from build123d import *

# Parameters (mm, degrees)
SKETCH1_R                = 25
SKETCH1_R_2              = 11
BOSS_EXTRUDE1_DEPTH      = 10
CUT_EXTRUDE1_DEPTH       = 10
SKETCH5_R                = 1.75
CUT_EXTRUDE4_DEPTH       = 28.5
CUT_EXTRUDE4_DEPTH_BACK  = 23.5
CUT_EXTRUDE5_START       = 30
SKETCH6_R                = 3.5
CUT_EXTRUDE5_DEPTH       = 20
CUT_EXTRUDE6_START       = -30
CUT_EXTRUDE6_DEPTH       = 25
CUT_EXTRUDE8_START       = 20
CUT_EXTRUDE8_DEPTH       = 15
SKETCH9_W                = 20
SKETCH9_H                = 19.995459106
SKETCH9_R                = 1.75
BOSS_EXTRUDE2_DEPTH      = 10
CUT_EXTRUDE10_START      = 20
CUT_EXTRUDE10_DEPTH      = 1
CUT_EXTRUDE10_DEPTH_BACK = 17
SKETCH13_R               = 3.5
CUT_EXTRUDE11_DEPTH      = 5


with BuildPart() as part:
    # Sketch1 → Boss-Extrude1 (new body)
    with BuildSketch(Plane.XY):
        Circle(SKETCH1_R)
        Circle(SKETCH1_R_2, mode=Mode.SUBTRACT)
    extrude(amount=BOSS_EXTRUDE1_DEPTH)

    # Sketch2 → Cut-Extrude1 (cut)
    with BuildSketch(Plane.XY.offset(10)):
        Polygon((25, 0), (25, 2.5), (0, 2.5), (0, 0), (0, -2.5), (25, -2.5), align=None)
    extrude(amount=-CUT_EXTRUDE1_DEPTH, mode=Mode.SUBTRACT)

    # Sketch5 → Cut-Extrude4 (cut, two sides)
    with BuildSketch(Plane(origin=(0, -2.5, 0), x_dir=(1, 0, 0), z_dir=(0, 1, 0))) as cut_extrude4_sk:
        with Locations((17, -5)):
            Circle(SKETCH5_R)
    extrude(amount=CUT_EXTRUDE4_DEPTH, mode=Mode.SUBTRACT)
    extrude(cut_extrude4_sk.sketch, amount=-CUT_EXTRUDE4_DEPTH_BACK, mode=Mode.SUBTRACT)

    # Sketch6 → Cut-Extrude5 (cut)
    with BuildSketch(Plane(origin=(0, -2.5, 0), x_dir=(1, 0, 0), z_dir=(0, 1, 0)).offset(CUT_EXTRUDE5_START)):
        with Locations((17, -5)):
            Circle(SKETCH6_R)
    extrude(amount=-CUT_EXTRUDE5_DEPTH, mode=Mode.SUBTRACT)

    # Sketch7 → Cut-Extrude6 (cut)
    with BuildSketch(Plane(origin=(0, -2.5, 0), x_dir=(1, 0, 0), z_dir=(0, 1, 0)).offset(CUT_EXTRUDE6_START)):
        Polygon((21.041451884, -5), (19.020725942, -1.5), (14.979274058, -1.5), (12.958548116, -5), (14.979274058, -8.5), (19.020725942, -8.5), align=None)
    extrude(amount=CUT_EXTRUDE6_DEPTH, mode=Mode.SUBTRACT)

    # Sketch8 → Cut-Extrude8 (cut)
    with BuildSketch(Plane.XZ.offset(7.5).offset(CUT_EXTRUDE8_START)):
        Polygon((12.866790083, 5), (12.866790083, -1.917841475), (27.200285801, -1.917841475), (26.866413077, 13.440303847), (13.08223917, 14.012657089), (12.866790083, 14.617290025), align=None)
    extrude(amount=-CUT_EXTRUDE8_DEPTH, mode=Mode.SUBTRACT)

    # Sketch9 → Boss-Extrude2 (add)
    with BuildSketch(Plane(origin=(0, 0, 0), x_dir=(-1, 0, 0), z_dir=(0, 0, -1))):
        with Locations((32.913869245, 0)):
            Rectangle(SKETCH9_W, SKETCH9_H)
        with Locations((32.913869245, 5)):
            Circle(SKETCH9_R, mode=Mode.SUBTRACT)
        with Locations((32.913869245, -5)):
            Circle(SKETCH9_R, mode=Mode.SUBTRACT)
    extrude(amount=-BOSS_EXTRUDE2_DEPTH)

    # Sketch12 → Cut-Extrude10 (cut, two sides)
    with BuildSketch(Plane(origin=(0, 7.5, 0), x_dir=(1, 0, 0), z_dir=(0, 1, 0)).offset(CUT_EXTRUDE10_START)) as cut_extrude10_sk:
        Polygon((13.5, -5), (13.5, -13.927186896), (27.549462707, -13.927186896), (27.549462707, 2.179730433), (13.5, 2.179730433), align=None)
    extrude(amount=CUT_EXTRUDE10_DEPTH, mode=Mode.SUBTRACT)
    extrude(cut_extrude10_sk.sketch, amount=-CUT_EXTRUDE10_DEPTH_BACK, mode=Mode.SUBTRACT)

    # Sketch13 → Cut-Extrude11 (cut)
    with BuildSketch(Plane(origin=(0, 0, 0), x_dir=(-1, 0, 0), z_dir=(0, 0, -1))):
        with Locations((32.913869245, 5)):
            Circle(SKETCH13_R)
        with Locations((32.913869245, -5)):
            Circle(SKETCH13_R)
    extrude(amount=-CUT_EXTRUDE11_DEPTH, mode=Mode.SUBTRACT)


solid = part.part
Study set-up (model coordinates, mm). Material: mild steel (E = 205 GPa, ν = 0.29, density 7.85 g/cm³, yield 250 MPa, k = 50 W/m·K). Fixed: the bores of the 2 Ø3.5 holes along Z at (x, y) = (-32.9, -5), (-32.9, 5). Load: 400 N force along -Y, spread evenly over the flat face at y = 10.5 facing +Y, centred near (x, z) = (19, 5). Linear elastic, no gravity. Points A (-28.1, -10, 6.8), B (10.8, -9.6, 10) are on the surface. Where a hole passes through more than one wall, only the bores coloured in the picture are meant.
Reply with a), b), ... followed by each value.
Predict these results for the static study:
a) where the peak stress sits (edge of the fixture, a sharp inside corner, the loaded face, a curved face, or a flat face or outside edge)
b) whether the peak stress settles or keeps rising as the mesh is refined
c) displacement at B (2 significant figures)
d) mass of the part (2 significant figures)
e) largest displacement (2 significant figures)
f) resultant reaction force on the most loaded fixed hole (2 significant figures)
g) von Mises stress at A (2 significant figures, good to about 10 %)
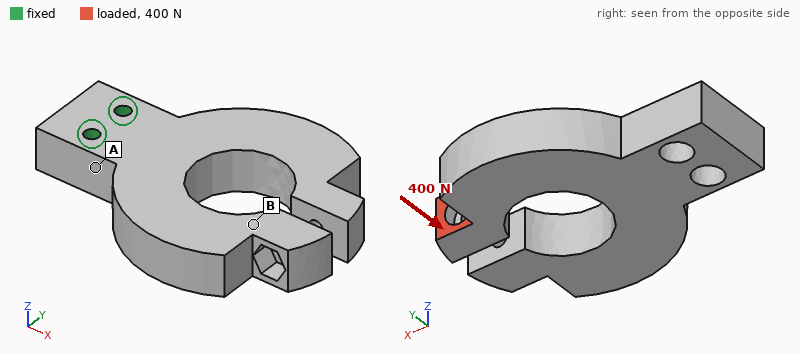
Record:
a) edge of the fixture
b) keeps rising
c) 12 µm
d) 130 g
e) 54 µm
f) 1.7 kN
g) 30 MPa
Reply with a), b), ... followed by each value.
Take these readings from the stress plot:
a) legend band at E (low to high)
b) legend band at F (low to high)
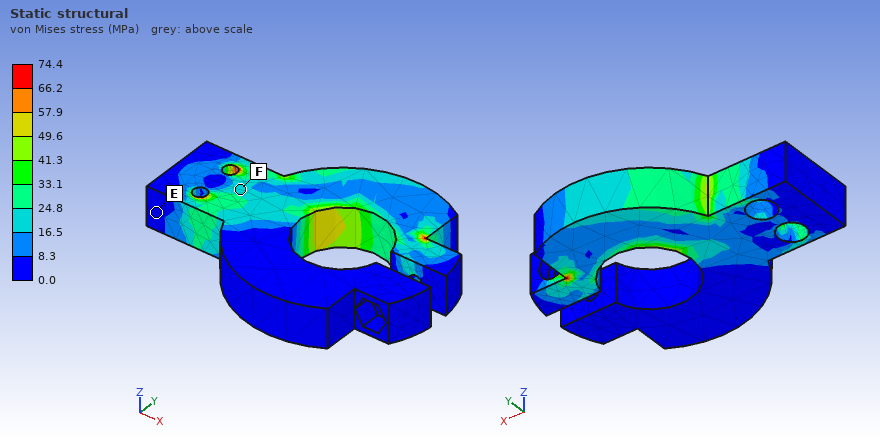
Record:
a) 0.0 to 8.3 MPa
b) 16.5 to 24.8 MPa
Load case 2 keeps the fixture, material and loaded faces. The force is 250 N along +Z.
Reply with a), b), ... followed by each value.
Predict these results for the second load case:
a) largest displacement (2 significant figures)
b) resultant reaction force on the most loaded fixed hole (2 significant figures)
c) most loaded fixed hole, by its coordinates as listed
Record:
a) 90 µm
b) 320 N
c) (-32.9, 5)
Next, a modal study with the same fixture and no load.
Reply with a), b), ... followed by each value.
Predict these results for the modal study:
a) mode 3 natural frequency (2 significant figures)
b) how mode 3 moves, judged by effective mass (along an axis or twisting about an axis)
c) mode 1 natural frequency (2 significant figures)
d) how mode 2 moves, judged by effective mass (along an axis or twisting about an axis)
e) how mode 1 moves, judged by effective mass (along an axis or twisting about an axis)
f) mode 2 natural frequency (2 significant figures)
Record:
a) 3300 Hz
b) along Y
c) 1700 Hz
d) along Y
e) along Z
f) 3100 Hz
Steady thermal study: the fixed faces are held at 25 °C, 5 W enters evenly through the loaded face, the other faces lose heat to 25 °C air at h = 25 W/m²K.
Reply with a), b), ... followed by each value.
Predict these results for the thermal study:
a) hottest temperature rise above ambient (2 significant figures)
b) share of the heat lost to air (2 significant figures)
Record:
a) 48 K
b) 34 %
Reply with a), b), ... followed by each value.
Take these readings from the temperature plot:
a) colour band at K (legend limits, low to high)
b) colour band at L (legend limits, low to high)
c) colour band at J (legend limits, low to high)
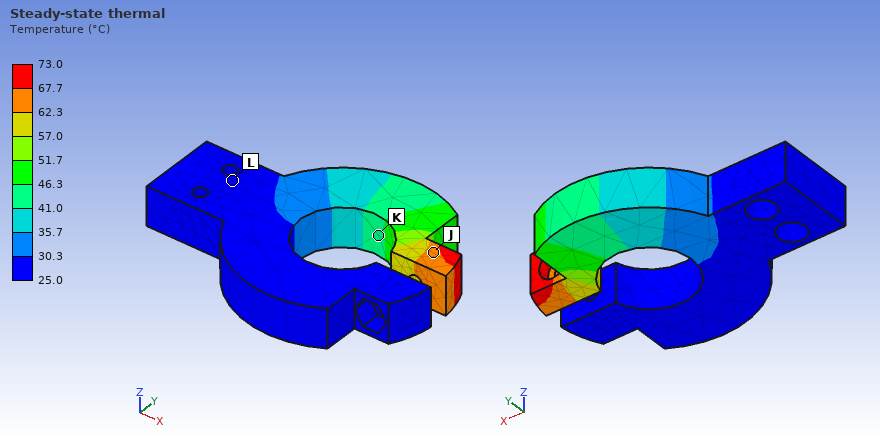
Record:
a) 41.0 to 46.3 °C
b) 25.0 to 30.3 °C
c) 62.3 to 67.7 °C
